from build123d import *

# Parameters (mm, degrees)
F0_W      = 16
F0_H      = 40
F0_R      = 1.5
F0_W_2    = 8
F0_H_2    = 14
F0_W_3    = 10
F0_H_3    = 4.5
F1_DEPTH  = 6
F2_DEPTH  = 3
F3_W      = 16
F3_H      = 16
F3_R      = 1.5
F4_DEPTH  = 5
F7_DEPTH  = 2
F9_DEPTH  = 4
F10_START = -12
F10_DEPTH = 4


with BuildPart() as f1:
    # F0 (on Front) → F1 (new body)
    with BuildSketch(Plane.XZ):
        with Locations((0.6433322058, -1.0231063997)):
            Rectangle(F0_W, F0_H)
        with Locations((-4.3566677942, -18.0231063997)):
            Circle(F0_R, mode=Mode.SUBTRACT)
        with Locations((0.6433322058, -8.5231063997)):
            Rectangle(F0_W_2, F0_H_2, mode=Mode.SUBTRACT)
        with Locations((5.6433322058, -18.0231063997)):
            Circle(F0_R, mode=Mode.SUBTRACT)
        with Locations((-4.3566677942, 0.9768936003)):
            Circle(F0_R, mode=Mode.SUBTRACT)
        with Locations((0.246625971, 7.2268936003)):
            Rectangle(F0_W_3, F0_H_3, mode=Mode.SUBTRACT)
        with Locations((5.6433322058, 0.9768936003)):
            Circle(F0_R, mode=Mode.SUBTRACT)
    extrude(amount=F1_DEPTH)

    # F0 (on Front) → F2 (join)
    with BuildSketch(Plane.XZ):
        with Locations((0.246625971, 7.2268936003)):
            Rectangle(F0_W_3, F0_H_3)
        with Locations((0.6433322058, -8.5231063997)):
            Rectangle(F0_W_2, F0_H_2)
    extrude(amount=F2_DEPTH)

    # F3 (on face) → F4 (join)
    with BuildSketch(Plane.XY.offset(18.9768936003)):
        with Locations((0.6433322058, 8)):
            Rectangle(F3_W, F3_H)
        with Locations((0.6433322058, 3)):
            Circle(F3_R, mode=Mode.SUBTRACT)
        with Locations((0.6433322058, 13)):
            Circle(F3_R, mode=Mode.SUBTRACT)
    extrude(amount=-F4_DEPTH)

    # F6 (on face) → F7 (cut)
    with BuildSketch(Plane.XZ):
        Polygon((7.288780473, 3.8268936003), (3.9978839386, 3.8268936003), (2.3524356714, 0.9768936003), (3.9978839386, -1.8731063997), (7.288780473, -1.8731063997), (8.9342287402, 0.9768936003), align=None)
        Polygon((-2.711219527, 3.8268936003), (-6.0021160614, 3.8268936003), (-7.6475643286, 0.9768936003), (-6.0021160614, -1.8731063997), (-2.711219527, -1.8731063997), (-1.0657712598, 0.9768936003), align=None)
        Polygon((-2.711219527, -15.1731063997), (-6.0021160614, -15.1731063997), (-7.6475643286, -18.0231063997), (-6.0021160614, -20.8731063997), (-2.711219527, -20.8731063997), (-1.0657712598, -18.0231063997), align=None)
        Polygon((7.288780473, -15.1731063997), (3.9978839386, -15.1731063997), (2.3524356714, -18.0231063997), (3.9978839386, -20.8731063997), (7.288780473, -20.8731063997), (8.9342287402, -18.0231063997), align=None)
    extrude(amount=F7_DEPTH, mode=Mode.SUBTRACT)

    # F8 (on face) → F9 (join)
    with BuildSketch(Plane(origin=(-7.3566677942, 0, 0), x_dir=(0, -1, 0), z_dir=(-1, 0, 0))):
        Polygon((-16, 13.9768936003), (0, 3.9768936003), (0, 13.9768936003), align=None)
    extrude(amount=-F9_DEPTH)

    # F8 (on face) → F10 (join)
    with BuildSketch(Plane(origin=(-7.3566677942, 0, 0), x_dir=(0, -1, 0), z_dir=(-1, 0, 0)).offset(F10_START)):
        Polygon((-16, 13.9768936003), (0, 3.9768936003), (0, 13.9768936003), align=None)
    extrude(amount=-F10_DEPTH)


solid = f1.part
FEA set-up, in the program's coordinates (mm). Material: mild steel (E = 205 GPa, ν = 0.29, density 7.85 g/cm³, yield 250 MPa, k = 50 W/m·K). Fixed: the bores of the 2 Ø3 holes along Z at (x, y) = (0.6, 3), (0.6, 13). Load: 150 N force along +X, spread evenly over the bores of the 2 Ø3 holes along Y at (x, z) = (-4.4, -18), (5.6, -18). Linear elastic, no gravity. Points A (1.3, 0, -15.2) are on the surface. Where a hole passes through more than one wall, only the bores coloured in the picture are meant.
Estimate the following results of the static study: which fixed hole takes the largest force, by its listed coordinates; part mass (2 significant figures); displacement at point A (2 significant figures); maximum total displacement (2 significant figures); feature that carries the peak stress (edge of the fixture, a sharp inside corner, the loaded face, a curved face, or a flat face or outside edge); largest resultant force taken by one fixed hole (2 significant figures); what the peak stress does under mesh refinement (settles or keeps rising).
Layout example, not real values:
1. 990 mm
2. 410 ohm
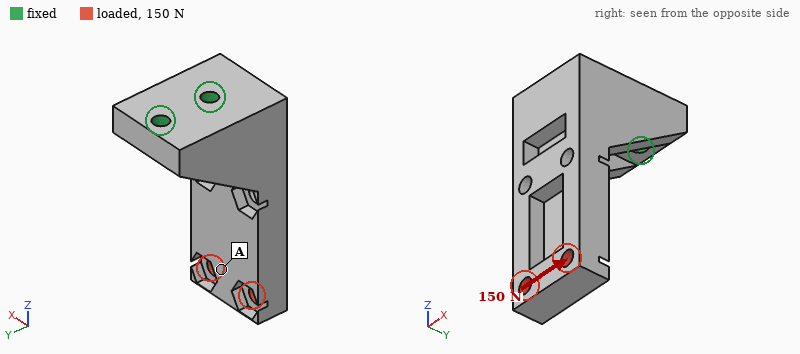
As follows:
1. (0.6, 3)
2. 38 g
3. 17 µm
4. 23 µm
5. edge of the fixture
6. 220 N
7. keeps rising
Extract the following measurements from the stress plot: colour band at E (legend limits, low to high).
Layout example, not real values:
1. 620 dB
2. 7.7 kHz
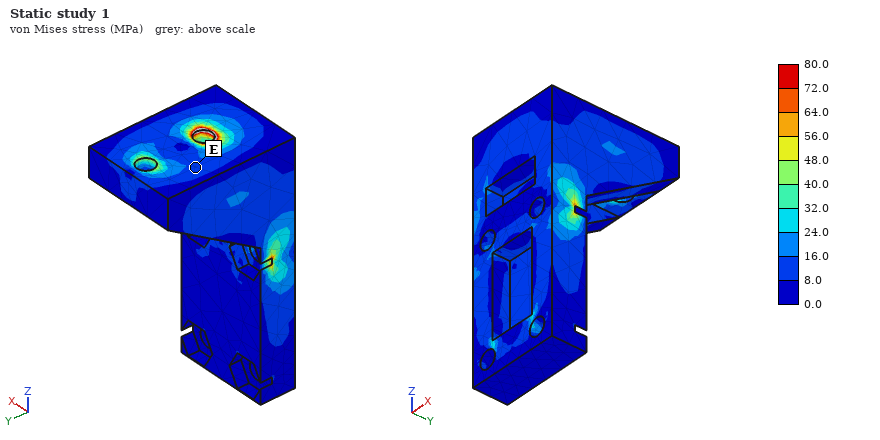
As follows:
1. 8.0 to 16.0 MPa
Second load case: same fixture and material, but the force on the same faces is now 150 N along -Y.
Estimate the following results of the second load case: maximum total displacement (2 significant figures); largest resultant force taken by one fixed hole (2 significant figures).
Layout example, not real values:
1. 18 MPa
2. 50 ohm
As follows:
1. 53 µm
2. 380 N
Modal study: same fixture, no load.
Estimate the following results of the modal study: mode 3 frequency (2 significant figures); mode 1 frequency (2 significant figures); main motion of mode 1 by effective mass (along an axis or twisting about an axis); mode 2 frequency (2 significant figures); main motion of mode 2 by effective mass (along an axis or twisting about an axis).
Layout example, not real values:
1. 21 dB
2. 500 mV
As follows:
1. 12 kHz
2. 3800 Hz
3. along Y
4. 5000 Hz
5. along X
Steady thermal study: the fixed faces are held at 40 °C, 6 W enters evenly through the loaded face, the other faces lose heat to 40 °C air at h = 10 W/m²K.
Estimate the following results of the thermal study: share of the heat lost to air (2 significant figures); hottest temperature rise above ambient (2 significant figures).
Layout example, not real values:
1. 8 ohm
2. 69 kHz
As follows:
1. 12 %
2. 62 K
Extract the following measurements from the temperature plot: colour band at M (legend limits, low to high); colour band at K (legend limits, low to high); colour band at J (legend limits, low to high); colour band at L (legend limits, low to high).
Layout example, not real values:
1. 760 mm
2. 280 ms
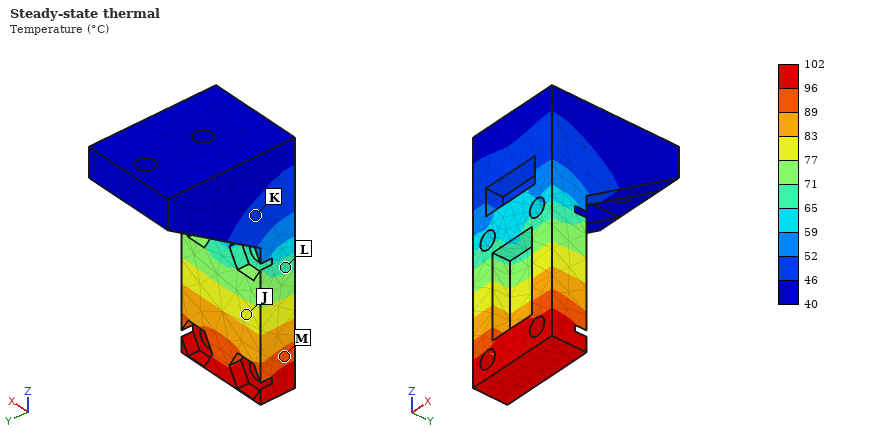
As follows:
1. 89 to 96 °C
2. 46 to 52 °C
3. 77 to 83 °C
4. 65 to 71 °C
